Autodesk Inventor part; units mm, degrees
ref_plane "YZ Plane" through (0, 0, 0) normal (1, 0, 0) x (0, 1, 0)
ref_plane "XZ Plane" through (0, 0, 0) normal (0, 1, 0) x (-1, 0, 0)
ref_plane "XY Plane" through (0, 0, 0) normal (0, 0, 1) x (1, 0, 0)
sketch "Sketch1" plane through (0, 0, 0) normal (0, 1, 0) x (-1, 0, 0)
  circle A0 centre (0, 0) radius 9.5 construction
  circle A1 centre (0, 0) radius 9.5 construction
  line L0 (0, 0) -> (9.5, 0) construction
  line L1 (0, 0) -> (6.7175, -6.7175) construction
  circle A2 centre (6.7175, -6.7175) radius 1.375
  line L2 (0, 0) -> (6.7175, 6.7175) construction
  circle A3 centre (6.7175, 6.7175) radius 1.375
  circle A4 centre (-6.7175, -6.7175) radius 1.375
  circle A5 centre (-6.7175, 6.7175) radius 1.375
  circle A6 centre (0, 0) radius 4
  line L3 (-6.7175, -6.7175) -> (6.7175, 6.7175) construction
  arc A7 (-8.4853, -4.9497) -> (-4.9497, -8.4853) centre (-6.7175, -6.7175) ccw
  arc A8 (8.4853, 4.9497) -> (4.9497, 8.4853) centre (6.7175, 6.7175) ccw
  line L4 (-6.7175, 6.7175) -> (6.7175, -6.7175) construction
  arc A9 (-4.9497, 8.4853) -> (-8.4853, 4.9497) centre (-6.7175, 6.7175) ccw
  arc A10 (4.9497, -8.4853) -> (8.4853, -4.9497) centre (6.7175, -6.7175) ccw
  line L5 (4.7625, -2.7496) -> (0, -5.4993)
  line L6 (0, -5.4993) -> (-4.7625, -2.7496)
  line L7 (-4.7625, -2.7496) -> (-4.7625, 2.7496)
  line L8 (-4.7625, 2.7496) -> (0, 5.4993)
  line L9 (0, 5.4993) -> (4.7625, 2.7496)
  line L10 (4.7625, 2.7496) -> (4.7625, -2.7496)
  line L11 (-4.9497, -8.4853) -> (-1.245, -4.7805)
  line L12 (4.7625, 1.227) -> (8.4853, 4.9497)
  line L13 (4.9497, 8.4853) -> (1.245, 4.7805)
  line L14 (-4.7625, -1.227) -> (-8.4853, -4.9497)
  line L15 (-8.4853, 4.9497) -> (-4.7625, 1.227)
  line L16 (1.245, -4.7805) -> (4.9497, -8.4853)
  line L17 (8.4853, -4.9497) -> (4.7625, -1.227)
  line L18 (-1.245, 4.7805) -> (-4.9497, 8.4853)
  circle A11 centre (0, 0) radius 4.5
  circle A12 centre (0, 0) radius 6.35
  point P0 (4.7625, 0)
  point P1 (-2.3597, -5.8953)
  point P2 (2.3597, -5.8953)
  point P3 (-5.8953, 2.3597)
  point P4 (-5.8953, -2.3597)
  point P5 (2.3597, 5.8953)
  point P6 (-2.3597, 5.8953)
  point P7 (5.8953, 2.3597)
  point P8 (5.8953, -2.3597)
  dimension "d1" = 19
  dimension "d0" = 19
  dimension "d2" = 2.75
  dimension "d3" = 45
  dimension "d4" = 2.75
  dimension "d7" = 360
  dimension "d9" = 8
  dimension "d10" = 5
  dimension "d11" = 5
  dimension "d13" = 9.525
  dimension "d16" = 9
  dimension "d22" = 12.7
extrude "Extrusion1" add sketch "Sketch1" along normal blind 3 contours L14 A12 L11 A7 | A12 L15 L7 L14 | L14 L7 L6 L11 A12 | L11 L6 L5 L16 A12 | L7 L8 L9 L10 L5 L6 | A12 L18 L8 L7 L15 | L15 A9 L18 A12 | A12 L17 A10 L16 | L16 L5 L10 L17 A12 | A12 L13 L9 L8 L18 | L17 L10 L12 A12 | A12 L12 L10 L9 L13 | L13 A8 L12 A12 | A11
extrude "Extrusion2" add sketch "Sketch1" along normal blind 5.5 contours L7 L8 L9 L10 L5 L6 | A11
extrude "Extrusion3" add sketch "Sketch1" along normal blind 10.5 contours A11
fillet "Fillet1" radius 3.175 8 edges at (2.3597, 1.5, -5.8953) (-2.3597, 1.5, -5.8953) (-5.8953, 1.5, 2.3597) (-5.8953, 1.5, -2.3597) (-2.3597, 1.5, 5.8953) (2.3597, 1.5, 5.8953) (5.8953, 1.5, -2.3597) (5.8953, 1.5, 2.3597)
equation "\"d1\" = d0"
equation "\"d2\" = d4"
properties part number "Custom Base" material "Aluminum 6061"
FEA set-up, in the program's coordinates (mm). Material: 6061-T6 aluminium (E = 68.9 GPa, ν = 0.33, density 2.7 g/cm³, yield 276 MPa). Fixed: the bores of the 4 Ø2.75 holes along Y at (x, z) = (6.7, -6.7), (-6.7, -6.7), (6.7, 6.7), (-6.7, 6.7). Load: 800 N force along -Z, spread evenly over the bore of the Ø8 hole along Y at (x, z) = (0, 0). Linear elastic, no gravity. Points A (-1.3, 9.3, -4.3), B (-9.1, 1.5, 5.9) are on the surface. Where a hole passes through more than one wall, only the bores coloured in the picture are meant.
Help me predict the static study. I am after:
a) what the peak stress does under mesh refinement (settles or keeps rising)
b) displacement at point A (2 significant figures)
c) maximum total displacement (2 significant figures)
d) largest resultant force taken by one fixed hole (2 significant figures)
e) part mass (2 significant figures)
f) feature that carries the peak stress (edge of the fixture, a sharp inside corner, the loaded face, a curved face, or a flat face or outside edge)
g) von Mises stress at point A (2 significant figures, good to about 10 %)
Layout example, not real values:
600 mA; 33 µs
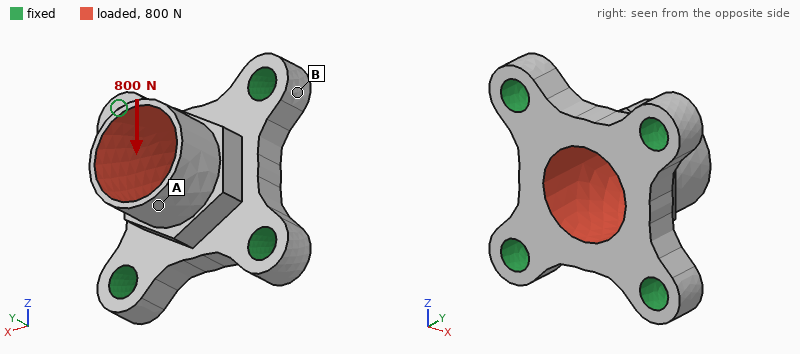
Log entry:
keeps rising; 19 µm; 21 µm; 260 N; 1.7 g; edge of the fixture; 29 MPa
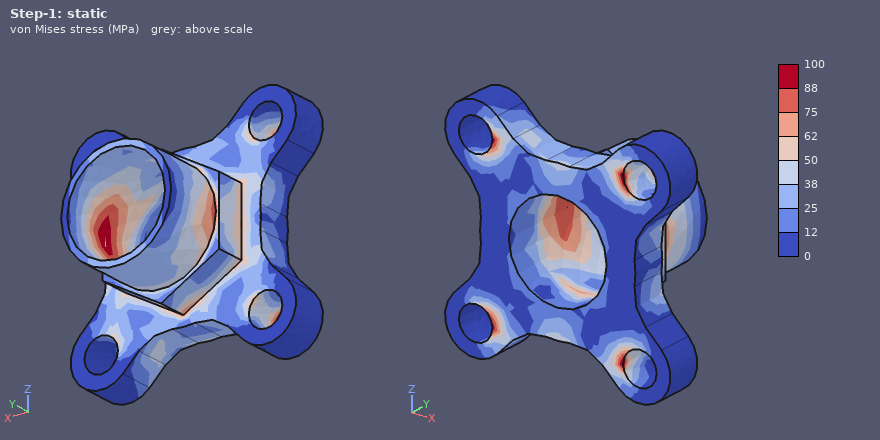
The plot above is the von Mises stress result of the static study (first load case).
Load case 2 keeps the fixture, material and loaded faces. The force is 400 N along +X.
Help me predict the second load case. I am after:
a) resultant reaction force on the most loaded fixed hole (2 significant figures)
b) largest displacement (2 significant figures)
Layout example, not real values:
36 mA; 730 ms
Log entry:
130 N; 10 µm
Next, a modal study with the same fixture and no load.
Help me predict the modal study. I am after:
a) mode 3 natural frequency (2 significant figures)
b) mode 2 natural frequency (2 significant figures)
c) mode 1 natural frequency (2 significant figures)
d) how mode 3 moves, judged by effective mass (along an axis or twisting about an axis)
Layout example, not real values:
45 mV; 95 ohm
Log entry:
54 kHz; 47 kHz; 42 kHz; along Z
